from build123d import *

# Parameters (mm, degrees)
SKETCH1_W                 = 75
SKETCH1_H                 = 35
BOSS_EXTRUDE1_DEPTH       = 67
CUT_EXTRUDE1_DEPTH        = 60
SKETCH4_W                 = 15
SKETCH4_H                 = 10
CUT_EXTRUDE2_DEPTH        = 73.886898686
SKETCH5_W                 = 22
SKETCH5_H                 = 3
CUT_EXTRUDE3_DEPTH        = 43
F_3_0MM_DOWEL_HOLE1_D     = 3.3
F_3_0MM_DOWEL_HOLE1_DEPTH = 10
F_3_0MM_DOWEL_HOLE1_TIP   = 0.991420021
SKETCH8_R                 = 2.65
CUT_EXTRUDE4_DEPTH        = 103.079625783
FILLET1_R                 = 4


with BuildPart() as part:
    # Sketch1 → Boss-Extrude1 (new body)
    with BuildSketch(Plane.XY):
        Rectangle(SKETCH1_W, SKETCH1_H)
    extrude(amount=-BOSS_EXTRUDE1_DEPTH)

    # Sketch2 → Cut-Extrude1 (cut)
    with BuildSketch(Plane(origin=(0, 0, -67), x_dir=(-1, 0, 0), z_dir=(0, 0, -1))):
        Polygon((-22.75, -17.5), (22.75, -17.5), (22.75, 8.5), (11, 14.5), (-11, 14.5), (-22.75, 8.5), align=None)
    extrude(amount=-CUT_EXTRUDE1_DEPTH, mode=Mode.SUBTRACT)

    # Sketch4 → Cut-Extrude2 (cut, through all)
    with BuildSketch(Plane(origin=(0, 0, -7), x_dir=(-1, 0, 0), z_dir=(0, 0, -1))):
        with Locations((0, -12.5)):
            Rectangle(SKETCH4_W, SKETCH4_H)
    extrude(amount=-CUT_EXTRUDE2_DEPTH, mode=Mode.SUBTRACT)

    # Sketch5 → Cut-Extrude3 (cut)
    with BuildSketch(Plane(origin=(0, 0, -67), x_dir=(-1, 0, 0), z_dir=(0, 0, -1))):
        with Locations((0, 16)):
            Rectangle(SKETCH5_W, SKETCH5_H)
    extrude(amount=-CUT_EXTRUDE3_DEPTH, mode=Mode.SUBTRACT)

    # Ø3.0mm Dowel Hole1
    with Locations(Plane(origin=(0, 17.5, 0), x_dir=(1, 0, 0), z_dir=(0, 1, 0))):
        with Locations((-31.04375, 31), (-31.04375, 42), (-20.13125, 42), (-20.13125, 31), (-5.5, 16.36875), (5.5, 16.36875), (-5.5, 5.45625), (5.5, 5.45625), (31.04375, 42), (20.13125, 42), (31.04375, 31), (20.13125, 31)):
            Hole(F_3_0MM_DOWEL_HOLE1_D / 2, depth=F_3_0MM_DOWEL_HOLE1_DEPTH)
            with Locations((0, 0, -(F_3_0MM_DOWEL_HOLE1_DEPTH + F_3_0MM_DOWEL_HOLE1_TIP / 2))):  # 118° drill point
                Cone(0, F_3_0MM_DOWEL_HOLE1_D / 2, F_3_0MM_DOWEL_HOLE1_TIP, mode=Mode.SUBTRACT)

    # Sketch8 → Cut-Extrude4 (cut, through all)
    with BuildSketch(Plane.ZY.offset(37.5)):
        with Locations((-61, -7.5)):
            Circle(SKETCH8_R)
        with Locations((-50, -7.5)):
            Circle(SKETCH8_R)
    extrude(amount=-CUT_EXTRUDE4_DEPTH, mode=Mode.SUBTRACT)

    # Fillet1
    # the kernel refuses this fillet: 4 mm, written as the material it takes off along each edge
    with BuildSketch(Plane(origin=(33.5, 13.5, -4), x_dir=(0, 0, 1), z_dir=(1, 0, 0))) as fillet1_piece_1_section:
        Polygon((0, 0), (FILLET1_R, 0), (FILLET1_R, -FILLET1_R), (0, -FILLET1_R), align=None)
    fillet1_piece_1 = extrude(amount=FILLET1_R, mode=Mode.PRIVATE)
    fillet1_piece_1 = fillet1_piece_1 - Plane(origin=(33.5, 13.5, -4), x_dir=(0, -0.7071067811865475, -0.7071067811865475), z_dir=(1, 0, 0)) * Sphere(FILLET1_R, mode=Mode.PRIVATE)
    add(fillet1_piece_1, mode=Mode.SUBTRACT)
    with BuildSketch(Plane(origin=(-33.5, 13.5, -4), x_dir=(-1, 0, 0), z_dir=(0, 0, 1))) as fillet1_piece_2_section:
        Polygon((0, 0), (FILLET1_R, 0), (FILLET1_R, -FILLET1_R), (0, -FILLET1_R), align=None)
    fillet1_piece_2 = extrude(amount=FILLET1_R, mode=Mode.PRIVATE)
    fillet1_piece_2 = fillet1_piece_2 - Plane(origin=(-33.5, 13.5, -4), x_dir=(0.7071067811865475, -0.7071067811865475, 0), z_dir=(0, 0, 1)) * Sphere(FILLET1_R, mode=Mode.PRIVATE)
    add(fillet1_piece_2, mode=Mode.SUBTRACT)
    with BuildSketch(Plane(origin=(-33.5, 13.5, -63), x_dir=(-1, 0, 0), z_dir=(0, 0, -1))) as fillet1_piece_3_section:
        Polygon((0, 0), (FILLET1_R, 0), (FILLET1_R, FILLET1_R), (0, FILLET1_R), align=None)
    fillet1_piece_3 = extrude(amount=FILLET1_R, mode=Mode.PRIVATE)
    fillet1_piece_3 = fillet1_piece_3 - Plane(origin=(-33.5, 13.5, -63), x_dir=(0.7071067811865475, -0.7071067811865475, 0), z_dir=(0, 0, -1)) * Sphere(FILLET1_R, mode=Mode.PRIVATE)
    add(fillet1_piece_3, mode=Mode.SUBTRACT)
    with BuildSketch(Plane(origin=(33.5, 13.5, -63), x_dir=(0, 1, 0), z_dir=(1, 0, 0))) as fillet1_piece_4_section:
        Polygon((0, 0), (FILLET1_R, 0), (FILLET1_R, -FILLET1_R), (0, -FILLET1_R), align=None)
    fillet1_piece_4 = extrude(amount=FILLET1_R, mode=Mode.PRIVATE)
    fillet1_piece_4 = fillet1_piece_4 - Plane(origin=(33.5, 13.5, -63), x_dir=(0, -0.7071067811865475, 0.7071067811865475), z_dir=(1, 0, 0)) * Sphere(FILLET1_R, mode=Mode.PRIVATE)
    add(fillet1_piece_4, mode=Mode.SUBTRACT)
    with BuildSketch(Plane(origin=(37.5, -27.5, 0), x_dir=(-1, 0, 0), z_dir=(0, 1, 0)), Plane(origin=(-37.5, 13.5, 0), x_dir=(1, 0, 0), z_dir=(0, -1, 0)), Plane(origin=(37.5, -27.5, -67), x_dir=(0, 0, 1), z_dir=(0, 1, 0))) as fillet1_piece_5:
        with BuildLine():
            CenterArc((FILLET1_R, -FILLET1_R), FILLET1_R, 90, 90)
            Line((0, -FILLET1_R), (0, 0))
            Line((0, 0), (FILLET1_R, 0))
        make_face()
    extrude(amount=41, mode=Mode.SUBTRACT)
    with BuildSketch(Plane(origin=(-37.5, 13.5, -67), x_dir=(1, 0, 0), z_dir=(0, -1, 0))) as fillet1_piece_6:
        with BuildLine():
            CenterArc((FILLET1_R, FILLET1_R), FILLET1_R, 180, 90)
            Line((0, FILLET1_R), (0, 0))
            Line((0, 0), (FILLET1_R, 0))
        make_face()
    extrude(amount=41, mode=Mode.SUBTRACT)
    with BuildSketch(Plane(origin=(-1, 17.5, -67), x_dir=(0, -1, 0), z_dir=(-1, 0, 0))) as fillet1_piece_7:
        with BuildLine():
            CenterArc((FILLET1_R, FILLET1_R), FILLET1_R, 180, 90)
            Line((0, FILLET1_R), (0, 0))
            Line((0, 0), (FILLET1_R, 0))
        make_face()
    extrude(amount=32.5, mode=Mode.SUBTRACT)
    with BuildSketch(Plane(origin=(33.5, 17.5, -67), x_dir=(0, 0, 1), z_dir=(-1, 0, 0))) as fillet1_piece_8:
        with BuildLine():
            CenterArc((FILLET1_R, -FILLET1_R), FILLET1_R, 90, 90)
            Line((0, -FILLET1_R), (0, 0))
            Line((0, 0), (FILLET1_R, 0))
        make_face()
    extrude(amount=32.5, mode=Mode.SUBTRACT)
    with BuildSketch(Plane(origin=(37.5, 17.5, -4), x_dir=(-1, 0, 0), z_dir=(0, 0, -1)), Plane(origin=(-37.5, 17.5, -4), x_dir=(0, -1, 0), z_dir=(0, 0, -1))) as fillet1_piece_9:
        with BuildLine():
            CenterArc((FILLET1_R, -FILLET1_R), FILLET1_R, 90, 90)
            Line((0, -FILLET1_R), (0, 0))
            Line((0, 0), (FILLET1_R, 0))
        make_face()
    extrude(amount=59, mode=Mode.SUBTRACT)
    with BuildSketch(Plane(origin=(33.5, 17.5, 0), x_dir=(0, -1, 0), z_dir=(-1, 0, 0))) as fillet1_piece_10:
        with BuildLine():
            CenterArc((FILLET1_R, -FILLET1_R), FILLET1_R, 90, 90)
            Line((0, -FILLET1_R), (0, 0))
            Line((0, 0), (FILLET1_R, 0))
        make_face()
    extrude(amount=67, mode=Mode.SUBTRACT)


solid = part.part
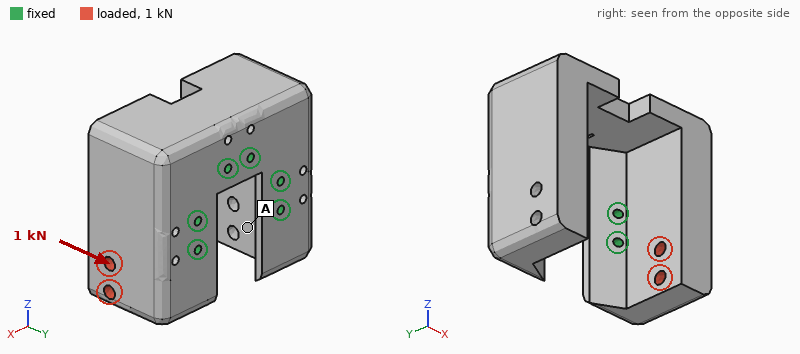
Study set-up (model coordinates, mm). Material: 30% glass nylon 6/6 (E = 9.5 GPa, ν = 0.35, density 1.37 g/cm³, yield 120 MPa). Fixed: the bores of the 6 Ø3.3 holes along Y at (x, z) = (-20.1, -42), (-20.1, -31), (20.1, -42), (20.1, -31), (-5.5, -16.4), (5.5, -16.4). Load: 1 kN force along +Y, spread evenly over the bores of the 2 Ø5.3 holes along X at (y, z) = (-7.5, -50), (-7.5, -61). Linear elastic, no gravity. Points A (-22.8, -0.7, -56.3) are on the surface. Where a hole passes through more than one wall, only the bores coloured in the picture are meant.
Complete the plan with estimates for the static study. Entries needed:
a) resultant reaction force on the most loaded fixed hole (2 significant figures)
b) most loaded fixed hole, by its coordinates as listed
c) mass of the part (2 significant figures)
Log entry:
1.2 kN
(20.1, -42)
120 g
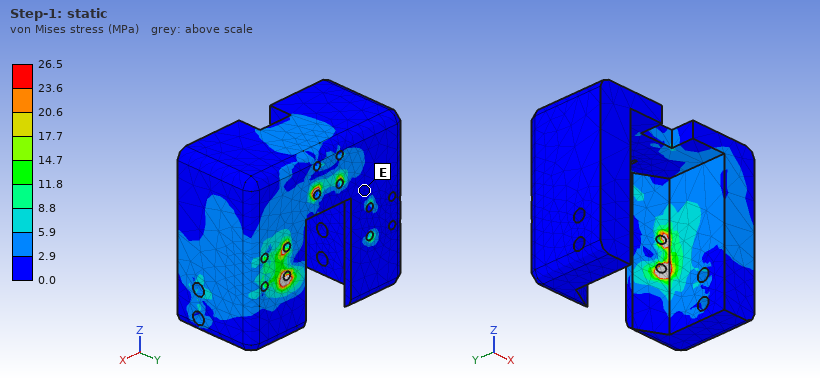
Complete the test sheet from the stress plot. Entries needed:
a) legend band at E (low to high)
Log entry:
0.0 to 2.9 MPa
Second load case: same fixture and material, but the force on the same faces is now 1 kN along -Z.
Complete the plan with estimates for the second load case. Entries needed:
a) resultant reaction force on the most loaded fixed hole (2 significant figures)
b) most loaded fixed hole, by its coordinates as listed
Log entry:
1.1 kN
(20.1, -42)
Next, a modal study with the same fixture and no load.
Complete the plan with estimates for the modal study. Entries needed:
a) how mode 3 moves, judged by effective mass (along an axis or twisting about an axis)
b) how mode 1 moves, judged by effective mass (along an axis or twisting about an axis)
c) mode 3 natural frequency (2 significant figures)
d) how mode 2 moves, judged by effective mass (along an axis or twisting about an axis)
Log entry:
along Y
along X
2600 Hz
along Z
